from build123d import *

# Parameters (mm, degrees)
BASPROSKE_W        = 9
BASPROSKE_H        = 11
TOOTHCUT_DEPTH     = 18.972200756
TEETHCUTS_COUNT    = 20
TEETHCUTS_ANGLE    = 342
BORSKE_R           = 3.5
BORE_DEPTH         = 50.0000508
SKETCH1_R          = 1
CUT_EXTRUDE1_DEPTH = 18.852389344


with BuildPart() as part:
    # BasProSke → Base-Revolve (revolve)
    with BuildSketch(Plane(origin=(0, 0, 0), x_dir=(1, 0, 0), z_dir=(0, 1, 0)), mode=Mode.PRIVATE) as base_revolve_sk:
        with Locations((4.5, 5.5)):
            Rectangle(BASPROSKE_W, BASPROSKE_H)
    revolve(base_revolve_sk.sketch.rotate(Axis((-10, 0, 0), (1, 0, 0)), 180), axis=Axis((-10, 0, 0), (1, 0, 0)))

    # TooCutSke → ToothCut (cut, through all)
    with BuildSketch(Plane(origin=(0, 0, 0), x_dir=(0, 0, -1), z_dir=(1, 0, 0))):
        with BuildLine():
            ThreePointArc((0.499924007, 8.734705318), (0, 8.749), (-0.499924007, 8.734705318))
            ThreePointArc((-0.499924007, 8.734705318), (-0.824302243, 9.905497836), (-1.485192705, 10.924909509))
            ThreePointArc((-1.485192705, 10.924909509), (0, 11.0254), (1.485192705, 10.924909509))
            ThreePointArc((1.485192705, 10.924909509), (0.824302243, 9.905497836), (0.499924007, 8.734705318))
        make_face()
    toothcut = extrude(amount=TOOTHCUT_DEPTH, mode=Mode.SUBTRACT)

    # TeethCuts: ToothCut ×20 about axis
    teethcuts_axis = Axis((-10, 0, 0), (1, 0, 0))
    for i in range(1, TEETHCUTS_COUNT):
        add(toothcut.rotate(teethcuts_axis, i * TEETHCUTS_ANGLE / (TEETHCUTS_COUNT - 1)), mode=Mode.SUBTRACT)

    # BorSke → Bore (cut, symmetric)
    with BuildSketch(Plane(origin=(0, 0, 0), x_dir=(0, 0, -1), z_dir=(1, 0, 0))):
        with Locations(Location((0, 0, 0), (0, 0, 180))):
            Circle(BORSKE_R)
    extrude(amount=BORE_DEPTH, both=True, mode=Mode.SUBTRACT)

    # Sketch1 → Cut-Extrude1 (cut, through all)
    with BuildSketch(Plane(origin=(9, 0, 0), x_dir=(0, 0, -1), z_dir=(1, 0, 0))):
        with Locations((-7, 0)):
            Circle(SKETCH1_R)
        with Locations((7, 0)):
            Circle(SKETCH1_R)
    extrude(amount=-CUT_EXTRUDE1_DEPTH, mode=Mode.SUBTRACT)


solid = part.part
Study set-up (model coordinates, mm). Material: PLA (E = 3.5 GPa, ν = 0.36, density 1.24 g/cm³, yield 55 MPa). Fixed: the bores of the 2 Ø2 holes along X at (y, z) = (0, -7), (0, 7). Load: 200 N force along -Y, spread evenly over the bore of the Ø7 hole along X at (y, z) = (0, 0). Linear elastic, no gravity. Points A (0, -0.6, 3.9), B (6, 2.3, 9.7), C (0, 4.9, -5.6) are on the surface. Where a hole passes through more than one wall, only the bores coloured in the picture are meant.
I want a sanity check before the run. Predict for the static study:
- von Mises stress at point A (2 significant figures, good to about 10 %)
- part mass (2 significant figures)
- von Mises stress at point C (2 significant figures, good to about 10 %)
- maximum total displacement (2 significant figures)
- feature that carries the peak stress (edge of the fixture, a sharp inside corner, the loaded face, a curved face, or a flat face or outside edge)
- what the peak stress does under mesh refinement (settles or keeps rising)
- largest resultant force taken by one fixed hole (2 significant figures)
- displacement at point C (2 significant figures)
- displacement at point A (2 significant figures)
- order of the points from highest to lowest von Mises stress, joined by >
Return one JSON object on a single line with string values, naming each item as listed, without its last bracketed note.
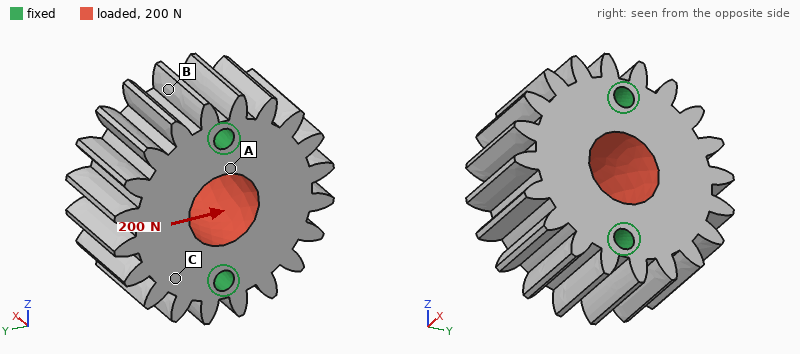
{"von Mises stress at point A": "1.7 MPa", "part mass": "2.9 g", "von Mises stress at point C": "0.99 MPa", "maximum total displacement": "4.6 µm", "feature that carries the peak stress": "edge of the fixture", "what the peak stress does under mesh refinement": "keeps rising", "largest resultant force taken by one fixed hole": "100 N", "displacement at point C": "2.0 µm", "displacement at point A": "2.8 µm", "order of the points from highest to lowest von Mises stress, joined by >": "A > C > B"}
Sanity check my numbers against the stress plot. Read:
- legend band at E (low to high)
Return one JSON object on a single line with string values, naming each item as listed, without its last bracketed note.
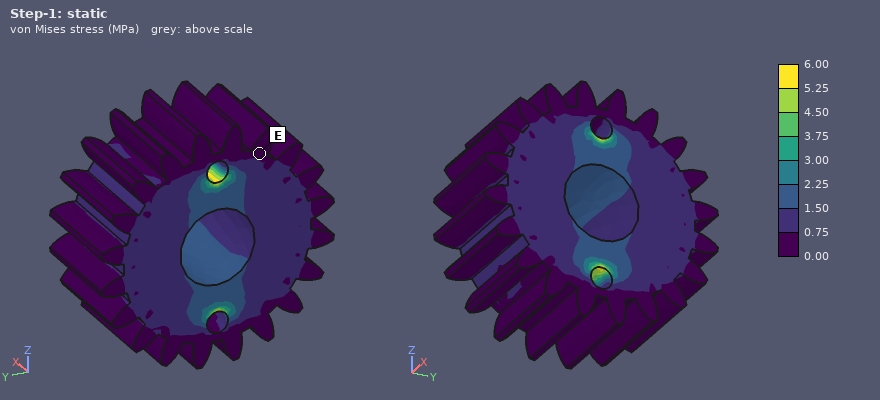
{"legend band at E": "0.00 to 0.75 MPa"}
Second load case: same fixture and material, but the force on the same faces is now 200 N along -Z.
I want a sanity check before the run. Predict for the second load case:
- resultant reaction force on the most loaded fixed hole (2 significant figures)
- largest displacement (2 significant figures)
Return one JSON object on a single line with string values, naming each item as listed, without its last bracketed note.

{"resultant reaction force on the most loaded fixed hole": "100 N", "largest displacement": "4.0 µm"}
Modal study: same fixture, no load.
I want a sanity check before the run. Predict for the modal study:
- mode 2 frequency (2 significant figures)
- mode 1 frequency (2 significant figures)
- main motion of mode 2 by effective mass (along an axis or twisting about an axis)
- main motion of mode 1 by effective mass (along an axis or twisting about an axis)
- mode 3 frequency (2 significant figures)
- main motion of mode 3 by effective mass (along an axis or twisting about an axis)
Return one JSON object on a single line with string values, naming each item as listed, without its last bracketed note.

{"mode 2 frequency": "16 kHz", "mode 1 frequency": "14 kHz", "main motion of mode 2 by effective mass": "along X", "main motion of mode 1 by effective mass": "twisting about Z", "mode 3 frequency": "21 kHz", "main motion of mode 3 by effective mass": "twisting about X"}
